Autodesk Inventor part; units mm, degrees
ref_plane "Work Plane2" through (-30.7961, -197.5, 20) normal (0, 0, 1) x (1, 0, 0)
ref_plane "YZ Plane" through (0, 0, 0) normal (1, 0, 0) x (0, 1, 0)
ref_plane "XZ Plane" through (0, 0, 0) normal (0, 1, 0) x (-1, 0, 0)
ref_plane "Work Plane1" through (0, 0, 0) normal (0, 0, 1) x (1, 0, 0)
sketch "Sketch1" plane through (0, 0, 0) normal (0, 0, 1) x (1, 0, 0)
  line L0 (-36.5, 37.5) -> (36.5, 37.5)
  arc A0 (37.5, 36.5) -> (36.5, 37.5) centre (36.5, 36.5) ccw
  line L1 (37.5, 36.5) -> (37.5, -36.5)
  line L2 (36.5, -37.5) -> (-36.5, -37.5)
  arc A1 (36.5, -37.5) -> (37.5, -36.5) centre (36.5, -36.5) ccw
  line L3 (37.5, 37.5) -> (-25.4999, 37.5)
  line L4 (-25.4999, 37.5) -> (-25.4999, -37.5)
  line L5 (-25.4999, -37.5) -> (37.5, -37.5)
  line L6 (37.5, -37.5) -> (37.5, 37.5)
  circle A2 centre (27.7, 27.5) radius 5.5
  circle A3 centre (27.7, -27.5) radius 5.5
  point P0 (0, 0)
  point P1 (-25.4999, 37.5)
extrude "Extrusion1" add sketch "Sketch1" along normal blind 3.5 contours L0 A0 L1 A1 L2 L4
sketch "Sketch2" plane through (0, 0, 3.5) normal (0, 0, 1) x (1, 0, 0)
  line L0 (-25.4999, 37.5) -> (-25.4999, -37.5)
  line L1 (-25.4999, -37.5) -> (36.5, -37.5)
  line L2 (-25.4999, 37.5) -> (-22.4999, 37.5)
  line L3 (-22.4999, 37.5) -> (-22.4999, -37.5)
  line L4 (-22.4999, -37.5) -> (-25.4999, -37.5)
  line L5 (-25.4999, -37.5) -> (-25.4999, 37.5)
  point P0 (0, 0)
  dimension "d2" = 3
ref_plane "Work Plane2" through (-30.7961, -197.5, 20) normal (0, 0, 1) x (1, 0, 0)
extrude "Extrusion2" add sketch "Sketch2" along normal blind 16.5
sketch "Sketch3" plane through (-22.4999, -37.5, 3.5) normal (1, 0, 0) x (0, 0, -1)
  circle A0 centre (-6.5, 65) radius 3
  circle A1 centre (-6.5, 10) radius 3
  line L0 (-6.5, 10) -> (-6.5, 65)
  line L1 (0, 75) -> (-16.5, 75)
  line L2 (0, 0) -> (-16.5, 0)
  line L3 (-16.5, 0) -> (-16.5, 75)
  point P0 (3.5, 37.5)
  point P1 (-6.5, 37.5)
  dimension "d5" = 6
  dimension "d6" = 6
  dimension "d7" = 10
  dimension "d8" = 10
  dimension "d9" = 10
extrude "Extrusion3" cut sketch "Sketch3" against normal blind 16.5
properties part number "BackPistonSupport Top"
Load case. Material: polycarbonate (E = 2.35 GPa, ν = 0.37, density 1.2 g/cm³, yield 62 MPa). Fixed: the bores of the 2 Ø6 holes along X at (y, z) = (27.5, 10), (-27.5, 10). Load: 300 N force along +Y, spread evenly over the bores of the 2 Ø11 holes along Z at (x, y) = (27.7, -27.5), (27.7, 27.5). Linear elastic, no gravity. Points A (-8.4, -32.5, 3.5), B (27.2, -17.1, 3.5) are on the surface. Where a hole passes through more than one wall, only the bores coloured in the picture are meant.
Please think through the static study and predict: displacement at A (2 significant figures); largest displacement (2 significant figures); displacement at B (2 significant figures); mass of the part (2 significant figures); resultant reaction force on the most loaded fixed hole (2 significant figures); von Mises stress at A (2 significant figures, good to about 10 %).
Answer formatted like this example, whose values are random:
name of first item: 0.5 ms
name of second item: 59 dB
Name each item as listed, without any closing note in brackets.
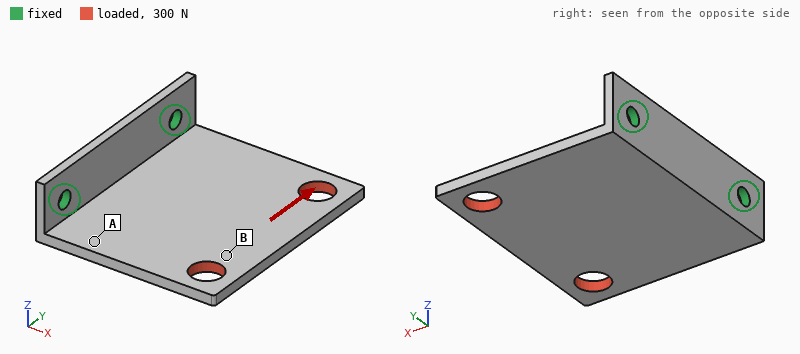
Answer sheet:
displacement at A: 0.52 mm
largest displacement: 1.2 mm
displacement at B: 0.71 mm
mass of the part: 23 g
resultant reaction force on the most loaded fixed hole: 320 N
von Mises stress at A: 7.3 MPa
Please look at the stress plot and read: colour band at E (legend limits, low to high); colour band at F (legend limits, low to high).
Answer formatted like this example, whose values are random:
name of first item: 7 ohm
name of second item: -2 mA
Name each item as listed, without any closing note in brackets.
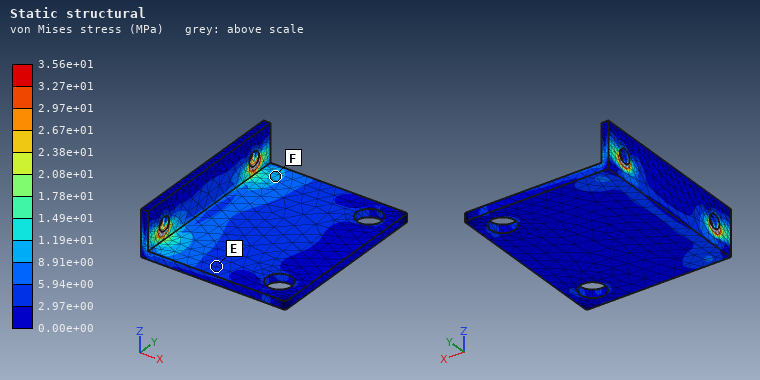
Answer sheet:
colour band at E: 2.97e+00 to 5.94e+00 MPa
colour band at F: 8.91e+00 to 1.19e+01 MPa
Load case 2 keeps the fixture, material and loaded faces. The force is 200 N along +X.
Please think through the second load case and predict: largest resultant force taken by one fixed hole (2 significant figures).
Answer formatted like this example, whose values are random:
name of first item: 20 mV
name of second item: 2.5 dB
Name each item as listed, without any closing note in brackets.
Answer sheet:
largest resultant force taken by one fixed hole: 100 N
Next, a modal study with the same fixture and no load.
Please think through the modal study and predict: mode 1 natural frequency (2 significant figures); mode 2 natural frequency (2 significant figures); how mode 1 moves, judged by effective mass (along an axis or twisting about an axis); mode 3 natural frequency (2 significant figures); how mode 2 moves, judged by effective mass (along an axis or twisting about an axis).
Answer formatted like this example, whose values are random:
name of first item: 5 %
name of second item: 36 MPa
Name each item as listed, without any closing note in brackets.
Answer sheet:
mode 1 natural frequency: 170 Hz
mode 2 natural frequency: 420 Hz
how mode 1 moves, judged by effective mass: along Z
mode 3 natural frequency: 1000 Hz
how mode 2 moves, judged by effective mass: twisting about X
